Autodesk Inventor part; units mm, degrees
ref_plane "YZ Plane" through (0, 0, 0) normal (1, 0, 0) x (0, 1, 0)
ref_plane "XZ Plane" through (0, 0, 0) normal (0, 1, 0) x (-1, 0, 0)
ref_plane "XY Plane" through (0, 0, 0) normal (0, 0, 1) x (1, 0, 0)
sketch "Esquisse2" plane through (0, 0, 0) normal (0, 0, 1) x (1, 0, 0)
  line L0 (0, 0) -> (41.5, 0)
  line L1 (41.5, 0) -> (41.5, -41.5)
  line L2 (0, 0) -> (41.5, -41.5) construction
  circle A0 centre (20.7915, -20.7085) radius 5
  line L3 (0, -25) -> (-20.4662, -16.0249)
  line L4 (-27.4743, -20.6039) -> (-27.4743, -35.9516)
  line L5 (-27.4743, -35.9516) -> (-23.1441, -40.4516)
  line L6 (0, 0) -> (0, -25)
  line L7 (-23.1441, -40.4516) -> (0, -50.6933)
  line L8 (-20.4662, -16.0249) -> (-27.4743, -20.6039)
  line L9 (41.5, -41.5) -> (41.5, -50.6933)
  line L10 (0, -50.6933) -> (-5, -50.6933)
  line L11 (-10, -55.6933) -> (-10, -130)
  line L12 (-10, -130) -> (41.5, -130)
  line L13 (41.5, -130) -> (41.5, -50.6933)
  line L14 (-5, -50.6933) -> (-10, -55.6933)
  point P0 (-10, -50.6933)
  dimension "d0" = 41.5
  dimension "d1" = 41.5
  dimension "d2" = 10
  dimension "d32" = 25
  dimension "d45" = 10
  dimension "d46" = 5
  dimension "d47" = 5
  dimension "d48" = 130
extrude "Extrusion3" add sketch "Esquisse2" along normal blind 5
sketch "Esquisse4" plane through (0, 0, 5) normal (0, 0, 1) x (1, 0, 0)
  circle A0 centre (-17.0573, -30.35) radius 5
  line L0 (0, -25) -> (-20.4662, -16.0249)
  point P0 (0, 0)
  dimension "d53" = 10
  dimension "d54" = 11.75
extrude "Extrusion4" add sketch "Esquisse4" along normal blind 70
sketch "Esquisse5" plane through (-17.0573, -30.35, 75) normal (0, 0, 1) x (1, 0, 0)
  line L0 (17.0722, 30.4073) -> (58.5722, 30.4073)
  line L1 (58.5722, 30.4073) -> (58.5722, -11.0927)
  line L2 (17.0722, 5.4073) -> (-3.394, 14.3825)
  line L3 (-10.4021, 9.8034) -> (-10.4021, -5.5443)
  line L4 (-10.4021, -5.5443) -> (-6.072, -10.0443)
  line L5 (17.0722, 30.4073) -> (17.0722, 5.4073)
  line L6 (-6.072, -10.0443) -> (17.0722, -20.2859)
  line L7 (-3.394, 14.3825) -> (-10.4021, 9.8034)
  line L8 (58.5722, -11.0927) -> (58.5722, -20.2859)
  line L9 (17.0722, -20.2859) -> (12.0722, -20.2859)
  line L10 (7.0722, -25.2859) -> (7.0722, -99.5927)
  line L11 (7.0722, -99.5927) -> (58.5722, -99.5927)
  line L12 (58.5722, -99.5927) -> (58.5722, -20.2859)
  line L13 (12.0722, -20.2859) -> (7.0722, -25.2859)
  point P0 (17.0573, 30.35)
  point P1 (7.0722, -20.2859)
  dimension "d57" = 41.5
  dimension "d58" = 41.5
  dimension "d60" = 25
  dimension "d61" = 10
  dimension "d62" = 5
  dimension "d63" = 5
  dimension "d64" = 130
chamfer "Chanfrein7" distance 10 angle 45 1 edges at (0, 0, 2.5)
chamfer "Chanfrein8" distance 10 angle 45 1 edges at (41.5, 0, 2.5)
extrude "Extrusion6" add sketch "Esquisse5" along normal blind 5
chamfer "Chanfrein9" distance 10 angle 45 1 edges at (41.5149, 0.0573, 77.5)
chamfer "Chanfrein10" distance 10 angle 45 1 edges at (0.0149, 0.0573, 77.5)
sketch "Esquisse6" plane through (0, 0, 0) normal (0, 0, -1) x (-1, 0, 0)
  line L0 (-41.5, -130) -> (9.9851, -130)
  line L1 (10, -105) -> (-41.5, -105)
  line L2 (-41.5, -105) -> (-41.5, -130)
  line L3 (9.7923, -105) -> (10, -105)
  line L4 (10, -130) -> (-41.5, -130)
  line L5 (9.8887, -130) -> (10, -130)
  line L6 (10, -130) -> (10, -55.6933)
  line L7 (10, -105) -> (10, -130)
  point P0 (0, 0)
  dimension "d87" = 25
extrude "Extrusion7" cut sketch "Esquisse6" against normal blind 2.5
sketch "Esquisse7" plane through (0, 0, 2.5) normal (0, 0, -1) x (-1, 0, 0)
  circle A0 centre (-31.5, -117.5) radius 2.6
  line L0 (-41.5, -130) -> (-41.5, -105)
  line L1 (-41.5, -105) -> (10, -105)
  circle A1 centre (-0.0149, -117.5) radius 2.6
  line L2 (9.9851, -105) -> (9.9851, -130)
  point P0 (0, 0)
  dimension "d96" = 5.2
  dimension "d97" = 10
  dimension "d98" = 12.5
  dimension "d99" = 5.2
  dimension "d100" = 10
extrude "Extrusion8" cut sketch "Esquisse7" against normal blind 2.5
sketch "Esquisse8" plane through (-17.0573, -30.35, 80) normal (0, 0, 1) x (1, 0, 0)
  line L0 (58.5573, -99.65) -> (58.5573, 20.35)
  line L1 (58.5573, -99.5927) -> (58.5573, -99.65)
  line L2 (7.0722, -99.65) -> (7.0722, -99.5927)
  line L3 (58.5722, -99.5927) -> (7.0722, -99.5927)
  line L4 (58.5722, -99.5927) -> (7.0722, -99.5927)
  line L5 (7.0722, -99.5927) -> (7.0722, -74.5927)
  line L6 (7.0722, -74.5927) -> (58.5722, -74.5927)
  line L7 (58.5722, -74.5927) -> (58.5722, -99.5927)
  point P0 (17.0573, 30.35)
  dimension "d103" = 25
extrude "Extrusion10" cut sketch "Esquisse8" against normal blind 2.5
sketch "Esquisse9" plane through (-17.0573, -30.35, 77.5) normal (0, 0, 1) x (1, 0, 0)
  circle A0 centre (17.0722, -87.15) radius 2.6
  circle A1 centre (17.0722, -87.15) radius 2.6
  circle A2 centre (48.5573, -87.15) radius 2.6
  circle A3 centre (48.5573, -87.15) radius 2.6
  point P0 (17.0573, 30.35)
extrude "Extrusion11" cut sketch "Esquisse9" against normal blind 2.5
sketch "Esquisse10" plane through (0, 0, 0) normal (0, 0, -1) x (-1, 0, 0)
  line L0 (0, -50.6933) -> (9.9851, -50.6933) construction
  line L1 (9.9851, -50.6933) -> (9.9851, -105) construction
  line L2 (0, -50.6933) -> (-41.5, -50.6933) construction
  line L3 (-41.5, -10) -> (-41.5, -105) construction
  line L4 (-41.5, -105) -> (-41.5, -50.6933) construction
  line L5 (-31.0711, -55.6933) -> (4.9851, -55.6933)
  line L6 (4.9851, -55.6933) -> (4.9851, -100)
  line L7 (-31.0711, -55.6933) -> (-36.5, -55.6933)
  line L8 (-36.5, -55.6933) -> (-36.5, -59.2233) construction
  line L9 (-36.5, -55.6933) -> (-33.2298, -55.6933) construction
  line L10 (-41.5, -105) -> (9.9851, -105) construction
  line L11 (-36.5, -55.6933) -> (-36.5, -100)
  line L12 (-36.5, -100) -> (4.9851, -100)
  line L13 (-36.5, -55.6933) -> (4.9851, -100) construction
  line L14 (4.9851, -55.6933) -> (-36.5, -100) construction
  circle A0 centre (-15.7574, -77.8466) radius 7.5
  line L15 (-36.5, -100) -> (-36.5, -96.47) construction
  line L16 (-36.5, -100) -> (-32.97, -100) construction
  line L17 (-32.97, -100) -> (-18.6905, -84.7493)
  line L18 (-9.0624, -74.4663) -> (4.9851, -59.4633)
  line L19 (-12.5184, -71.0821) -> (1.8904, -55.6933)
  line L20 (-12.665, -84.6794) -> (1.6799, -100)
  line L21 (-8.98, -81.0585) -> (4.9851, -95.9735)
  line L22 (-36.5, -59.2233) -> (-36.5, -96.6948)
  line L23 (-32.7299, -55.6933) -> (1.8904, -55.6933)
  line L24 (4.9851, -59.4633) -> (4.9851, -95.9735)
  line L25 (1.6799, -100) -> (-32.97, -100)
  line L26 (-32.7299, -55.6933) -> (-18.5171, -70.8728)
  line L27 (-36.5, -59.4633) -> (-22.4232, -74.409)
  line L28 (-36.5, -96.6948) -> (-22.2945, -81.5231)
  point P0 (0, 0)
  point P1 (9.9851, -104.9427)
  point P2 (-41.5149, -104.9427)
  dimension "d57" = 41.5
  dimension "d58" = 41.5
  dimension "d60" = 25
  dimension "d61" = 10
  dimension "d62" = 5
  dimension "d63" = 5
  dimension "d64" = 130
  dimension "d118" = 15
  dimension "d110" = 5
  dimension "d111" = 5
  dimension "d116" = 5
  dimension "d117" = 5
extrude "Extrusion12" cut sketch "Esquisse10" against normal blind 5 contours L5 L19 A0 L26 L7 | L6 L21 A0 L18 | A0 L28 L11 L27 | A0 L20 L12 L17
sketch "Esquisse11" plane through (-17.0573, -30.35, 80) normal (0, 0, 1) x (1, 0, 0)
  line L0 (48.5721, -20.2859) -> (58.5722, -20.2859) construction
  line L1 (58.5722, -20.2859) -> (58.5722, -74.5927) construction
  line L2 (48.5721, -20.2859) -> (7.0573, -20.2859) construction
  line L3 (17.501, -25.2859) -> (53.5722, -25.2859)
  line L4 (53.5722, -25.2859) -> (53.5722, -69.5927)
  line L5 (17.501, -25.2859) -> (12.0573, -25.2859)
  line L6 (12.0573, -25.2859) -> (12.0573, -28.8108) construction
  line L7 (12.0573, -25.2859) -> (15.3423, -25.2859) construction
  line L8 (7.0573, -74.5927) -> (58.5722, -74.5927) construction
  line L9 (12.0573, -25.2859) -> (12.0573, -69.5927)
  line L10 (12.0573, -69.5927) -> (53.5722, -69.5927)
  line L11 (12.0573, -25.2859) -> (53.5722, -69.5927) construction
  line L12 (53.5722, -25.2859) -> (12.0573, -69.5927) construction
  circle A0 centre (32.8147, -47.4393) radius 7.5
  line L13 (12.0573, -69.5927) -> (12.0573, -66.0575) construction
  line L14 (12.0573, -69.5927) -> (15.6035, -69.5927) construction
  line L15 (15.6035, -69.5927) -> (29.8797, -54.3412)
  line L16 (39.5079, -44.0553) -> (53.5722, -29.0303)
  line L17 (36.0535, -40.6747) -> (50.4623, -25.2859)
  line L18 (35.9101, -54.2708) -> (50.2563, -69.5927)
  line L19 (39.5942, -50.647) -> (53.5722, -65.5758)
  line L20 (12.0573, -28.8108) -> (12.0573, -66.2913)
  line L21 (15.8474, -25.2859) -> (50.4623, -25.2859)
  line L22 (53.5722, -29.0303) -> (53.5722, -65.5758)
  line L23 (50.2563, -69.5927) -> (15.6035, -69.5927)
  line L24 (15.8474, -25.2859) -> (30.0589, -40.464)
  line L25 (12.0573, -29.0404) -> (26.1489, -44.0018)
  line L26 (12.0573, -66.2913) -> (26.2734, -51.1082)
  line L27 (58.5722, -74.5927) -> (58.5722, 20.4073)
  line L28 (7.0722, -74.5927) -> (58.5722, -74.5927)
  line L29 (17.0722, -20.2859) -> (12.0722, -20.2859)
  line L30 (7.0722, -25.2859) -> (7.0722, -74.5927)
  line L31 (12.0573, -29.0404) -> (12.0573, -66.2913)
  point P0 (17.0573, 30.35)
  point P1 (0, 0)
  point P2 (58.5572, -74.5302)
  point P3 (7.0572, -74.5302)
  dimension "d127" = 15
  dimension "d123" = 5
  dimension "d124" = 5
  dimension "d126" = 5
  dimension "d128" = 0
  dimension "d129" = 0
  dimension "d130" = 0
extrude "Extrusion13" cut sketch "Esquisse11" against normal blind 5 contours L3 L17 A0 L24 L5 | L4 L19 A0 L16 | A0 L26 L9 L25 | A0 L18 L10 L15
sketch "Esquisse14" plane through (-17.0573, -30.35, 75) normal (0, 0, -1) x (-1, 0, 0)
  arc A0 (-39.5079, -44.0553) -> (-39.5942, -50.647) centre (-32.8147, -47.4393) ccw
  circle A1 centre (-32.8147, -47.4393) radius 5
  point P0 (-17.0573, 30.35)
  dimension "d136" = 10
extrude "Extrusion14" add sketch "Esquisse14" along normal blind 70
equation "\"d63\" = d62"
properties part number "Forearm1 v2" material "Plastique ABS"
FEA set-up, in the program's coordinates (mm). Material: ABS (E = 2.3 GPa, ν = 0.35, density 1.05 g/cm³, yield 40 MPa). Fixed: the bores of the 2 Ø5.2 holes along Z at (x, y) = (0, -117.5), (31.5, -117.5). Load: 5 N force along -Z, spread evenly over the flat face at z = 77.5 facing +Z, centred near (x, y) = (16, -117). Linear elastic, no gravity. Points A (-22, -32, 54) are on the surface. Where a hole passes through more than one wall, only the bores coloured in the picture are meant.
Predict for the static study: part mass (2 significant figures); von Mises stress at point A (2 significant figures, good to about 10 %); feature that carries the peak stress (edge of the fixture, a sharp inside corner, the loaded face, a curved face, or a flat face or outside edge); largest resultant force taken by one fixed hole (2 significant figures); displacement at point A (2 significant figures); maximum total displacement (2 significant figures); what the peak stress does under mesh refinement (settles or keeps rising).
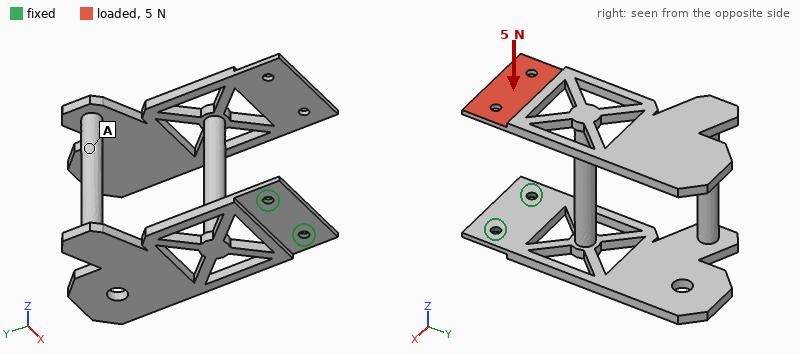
62 g
0.33 MPa
a sharp inside corner
2.5 N
1.2 mm
1.9 mm
keeps rising
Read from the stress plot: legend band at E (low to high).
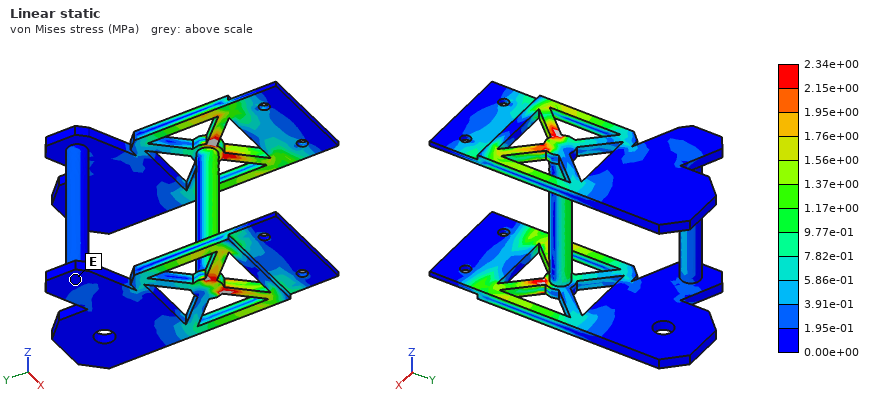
0.00e+00 to 1.95e-01 MPa
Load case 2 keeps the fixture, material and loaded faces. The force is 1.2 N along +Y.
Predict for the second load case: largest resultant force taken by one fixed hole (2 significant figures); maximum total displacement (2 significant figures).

0.62 N
1.9 mm
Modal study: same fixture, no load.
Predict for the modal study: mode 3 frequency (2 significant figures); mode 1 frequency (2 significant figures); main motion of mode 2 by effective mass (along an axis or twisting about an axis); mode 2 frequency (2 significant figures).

120 Hz
21 Hz
along X
42 Hz
